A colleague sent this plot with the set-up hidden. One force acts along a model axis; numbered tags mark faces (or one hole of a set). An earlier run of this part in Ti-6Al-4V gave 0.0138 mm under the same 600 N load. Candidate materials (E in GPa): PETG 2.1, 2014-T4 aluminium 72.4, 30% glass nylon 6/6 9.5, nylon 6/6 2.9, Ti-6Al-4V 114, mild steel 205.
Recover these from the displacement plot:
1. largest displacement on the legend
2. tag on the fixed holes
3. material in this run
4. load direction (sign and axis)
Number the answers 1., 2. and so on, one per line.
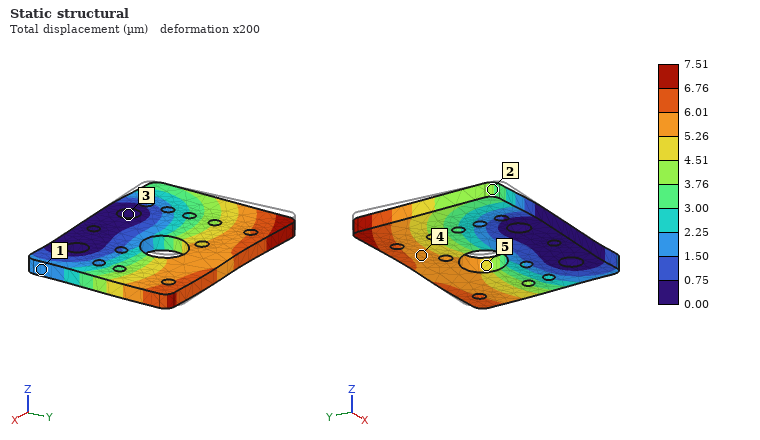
1. 7.51 µm
2. 3
3. mild steel
4. +X
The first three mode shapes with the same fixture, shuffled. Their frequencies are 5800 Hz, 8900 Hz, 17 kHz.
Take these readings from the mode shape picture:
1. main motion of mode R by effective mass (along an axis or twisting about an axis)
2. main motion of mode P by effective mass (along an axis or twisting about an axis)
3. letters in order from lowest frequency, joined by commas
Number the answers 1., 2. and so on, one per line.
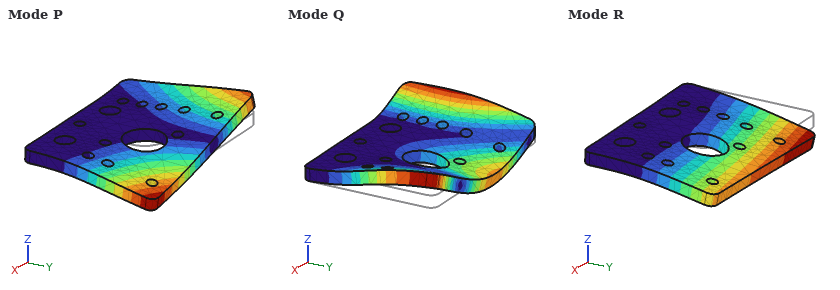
1. along Z
2. twisting about Y
3. R, P, Q
